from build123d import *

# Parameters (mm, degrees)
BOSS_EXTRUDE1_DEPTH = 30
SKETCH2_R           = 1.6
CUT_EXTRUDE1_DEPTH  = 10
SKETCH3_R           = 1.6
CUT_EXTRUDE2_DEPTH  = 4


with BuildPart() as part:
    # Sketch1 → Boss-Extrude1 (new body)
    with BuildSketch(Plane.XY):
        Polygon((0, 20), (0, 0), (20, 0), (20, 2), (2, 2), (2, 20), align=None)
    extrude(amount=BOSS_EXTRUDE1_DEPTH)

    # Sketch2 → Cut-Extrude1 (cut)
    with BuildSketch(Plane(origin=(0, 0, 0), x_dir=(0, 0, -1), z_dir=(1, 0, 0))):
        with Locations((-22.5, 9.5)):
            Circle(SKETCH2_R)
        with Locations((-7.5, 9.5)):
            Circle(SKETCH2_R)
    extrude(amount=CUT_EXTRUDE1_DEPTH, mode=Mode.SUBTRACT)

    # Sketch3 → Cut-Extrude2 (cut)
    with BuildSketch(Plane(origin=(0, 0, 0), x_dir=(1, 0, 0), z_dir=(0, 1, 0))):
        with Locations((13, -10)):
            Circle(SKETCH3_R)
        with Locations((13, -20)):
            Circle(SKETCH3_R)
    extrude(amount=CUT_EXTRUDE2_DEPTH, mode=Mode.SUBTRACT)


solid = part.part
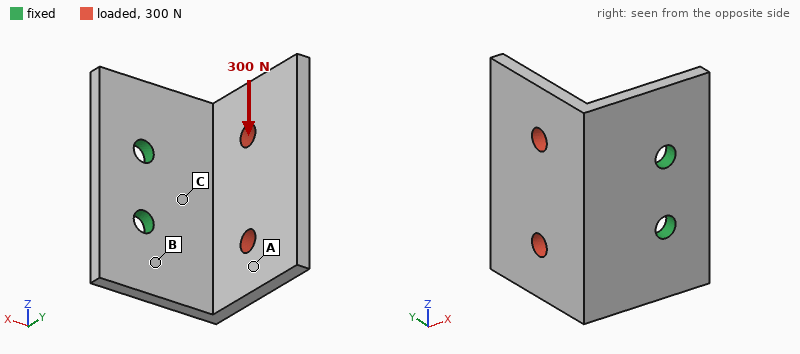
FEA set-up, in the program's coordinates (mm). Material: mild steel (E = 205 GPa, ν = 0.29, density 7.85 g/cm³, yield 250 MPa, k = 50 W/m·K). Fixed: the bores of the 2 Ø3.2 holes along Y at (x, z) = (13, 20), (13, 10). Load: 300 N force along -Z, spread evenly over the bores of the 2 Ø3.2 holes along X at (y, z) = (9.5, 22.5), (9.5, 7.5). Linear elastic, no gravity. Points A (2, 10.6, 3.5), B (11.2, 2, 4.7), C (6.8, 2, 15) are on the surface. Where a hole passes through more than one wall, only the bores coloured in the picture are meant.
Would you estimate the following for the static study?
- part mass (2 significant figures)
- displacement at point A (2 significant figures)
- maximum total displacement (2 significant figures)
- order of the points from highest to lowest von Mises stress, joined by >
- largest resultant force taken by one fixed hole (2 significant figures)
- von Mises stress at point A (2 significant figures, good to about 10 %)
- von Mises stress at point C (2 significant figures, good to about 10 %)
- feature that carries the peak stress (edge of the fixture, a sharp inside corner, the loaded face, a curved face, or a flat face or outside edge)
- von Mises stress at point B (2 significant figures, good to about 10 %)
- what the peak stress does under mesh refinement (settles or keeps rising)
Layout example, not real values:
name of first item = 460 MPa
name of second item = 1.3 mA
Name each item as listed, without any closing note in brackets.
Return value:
part mass = 17 g
displacement at point A = 36 µm
maximum total displacement = 58 µm
order of the points from highest to lowest von Mises stress, joined by > = C > B > A
largest resultant force taken by one fixed hole = 350 N
von Mises stress at point A = 21 MPa
von Mises stress at point C = 84 MPa
feature that carries the peak stress = edge of the fixture
von Mises stress at point B = 54 MPa
what the peak stress does under mesh refinement = keeps rising
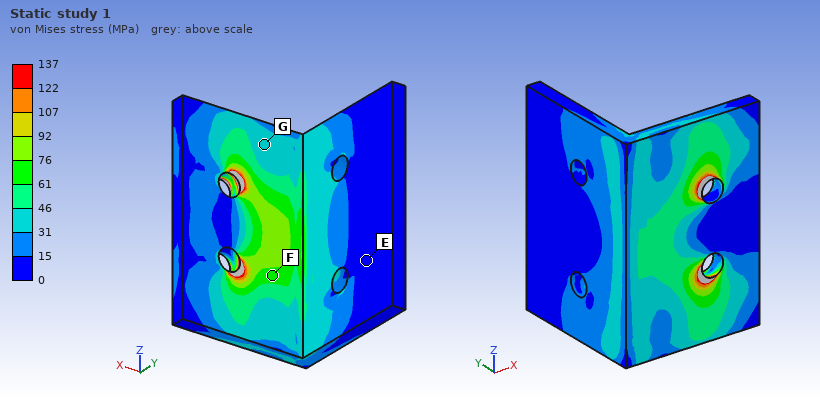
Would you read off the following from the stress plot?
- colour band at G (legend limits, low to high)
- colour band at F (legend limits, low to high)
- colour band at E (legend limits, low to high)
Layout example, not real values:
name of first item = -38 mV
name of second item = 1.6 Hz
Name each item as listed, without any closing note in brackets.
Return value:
colour band at G = 31 to 46 MPa
colour band at F = 61 to 76 MPa
colour band at E = 0 to 15 MPa
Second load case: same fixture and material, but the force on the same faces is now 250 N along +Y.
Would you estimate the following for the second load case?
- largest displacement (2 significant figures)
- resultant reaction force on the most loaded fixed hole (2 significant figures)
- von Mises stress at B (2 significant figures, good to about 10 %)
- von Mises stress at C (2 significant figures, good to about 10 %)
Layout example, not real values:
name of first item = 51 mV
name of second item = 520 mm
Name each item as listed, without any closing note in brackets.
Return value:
largest displacement = 87 µm
resultant reaction force on the most loaded fixed hole = 130 N
von Mises stress at B = 74 MPa
von Mises stress at C = 76 MPa
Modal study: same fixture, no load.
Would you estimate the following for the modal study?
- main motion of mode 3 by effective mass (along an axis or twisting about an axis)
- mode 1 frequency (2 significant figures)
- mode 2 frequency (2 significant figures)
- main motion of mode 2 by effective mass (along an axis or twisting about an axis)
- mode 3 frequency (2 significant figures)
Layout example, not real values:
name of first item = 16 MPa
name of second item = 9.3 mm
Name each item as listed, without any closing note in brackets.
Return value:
main motion of mode 3 by effective mass = along Y
mode 1 frequency = 2300 Hz
mode 2 frequency = 3800 Hz
main motion of mode 2 by effective mass = along Z
mode 3 frequency = 6800 Hz
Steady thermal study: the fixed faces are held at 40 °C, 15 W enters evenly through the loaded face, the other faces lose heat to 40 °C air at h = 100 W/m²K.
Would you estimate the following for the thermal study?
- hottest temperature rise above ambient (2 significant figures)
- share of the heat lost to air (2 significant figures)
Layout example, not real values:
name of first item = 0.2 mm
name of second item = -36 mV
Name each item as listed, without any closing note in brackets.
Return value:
hottest temperature rise above ambient = 68 K
share of the heat lost to air = 52 %
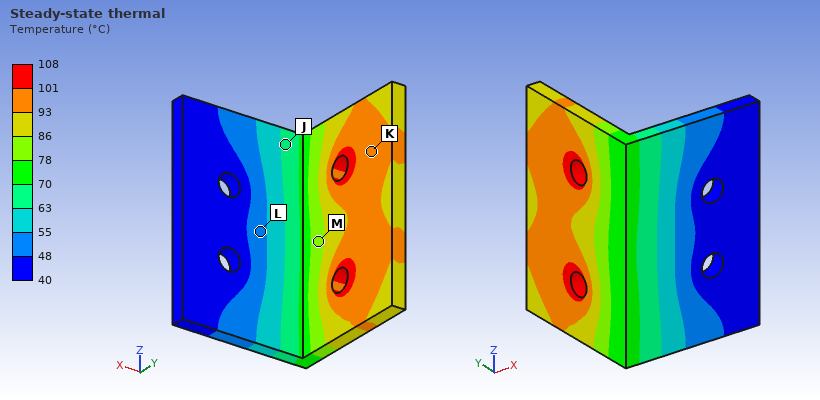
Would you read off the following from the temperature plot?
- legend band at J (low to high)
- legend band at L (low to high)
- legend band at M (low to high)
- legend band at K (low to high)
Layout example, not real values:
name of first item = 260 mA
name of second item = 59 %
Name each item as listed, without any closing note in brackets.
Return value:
legend band at J = 63 to 70 °C
legend band at L = 48 to 55 °C
legend band at M = 78 to 86 °C
legend band at K = 93 to 101 °C
